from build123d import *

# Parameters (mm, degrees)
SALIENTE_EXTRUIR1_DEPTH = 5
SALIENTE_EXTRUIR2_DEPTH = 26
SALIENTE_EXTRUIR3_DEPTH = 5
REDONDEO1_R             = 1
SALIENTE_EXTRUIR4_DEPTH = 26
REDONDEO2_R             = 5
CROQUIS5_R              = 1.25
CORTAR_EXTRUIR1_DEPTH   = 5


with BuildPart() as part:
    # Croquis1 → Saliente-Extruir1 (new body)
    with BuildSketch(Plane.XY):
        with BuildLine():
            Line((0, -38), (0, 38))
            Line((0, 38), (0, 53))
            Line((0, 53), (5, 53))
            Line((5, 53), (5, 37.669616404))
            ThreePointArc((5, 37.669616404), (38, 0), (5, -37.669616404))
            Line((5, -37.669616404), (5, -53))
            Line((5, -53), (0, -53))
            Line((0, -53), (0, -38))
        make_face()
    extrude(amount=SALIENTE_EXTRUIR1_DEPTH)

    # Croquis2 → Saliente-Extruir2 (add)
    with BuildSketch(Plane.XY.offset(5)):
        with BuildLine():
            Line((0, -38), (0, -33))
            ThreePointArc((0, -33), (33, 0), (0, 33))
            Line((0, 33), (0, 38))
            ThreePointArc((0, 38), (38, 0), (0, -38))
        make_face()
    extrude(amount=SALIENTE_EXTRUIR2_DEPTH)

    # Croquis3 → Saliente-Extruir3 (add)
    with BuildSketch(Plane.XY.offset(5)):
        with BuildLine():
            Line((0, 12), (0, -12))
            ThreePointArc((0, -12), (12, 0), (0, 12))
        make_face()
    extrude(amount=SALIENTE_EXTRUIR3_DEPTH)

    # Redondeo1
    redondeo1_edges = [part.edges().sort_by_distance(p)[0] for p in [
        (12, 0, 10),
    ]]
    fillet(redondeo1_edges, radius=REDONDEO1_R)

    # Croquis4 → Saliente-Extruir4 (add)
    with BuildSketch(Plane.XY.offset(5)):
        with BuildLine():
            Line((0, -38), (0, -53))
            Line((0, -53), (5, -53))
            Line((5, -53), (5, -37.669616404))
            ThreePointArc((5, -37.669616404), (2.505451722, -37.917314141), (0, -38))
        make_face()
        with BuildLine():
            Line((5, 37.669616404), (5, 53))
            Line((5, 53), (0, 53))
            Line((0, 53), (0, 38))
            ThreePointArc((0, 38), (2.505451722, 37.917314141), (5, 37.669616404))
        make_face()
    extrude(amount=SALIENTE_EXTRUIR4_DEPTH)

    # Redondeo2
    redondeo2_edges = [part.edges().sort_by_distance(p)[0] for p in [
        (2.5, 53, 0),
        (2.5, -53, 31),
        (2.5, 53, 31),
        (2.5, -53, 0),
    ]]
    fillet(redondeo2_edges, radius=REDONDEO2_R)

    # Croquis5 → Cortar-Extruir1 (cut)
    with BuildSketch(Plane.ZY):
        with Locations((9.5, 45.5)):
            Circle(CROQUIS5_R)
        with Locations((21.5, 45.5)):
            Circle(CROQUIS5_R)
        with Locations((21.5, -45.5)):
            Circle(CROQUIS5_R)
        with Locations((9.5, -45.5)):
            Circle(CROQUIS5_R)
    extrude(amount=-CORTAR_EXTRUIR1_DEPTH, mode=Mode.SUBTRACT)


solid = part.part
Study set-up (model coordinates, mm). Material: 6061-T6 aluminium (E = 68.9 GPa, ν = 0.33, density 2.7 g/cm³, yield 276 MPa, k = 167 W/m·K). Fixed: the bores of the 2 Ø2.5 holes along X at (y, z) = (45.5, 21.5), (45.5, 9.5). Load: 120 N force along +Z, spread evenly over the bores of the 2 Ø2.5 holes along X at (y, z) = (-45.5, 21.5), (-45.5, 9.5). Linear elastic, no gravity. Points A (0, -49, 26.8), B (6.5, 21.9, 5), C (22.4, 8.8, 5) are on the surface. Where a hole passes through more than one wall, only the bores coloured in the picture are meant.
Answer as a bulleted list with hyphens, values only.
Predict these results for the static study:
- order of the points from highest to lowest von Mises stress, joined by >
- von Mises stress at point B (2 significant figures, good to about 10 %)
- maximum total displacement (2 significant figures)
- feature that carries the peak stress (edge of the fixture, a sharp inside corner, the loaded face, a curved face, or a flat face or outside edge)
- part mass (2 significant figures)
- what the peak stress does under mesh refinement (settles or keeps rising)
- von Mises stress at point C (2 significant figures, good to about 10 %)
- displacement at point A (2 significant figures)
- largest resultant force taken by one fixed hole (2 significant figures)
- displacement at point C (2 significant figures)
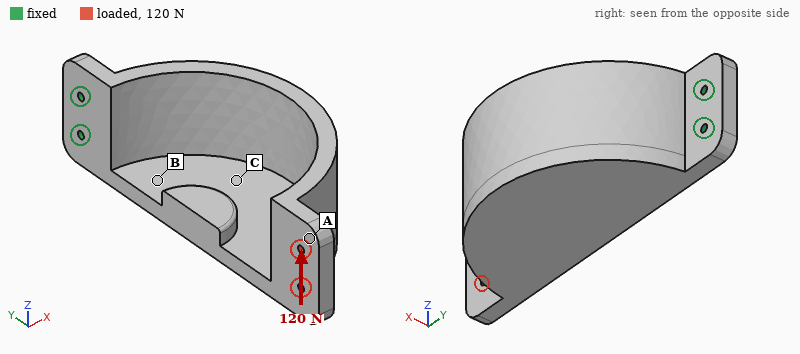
- B > C > A
- 26 MPa
- 0.49 mm
- edge of the fixture
- 85 g
- keeps rising
- 14 MPa
- 0.47 mm
- 810 N
- 0.093 mm
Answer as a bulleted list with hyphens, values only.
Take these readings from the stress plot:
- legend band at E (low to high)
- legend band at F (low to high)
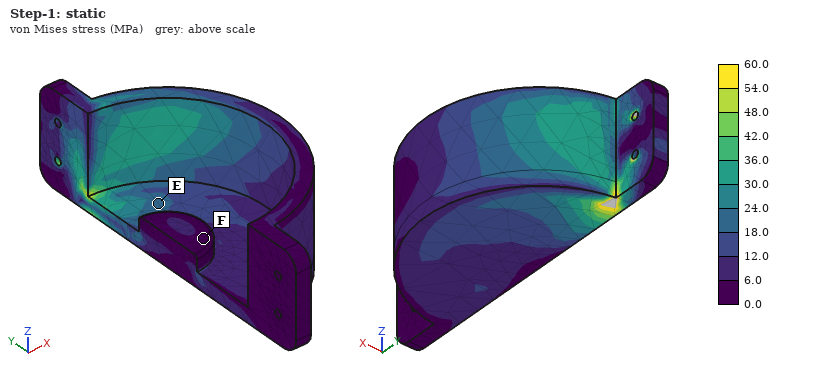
- 18.0 to 24.0 MPa
- 0.0 to 6.0 MPa
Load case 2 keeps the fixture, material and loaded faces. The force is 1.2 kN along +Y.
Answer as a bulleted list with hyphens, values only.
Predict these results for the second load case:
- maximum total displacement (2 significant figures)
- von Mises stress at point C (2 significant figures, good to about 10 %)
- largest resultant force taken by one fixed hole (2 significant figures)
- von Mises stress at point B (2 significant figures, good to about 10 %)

- 0.93 mm
- 22 MPa
- 610 N
- 54 MPa
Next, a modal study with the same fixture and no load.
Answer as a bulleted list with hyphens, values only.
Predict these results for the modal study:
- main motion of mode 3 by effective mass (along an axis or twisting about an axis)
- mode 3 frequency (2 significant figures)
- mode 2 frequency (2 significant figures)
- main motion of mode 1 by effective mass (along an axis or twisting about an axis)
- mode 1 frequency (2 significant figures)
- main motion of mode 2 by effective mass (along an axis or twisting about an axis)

- along Z
- 2000 Hz
- 620 Hz
- along X
- 380 Hz
- along Z
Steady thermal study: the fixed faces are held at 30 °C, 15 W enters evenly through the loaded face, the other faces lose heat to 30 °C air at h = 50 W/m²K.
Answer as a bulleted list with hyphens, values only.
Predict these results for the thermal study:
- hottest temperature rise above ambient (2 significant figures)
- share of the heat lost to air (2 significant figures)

- 30 K
- 56 %
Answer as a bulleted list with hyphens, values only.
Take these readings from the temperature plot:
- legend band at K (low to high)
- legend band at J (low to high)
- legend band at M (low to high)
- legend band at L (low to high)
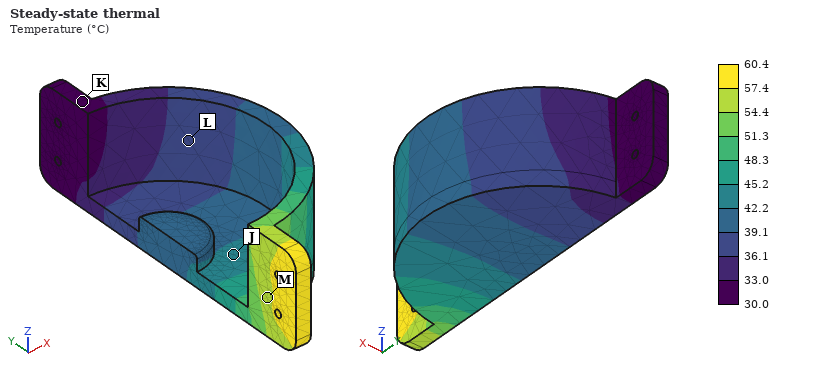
- 30.0 to 33.0 °C
- 42.2 to 45.2 °C
- 54.4 to 57.4 °C
- 36.1 to 39.1 °C
